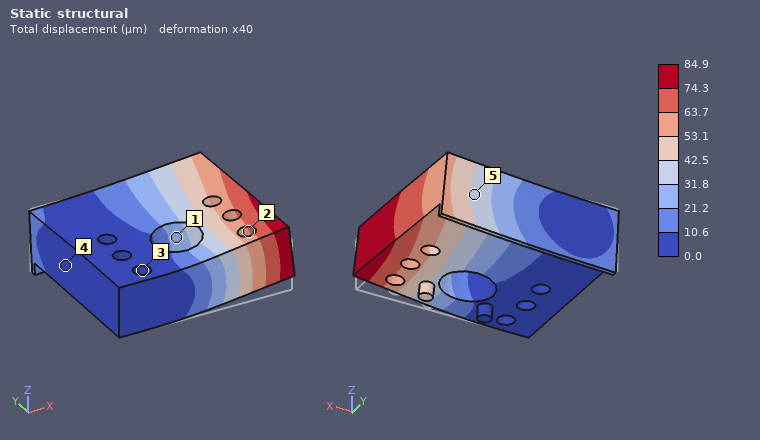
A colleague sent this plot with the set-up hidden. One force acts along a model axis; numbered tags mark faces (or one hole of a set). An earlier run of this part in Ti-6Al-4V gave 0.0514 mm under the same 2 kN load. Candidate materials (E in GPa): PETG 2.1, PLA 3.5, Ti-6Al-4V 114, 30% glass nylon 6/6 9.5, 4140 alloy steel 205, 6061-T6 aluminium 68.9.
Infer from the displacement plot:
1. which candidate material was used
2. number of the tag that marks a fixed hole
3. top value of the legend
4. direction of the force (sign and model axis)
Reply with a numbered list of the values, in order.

1. 6061-T6 aluminium
2. 3
3. 84.9 µm
4. +Z
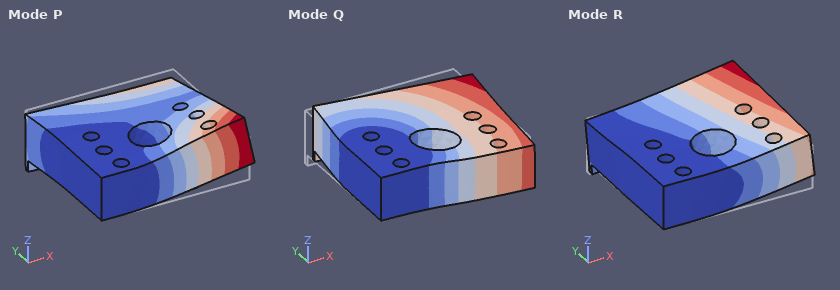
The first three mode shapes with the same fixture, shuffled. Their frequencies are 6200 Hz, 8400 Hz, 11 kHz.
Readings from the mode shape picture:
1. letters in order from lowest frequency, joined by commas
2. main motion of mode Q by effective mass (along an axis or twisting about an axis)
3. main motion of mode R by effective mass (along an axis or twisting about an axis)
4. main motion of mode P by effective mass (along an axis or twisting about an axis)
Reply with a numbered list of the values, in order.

1. R, Q, P
2. along Y
3. along Z
4. twisting about X
